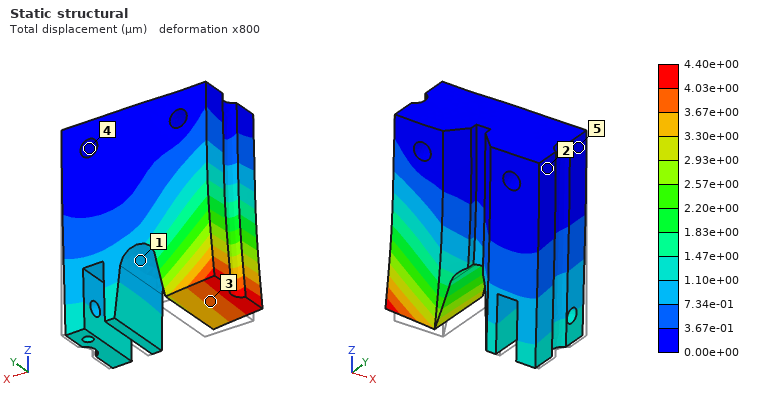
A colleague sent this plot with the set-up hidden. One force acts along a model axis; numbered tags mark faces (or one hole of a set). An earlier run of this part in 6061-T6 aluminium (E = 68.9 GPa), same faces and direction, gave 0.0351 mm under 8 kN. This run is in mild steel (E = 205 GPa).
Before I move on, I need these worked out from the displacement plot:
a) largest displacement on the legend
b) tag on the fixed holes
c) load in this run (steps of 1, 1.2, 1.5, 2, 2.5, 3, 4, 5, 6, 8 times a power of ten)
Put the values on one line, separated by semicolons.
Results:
4.40e+00 µm; 4; 3 kN
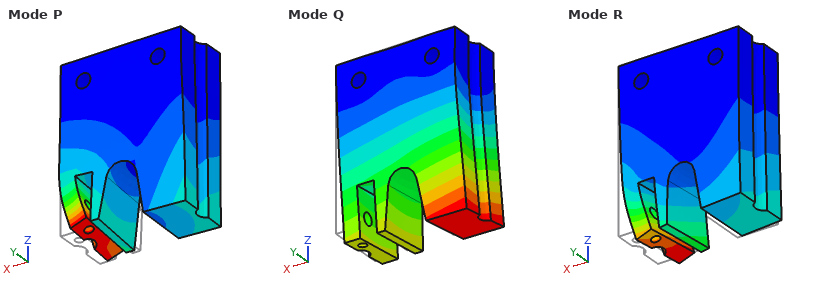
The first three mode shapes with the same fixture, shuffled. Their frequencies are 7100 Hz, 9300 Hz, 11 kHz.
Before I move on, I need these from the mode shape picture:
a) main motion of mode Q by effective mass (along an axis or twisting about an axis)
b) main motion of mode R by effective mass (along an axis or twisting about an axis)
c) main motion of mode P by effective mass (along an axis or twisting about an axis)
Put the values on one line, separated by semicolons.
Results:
along Y; along X; twisting about Z
